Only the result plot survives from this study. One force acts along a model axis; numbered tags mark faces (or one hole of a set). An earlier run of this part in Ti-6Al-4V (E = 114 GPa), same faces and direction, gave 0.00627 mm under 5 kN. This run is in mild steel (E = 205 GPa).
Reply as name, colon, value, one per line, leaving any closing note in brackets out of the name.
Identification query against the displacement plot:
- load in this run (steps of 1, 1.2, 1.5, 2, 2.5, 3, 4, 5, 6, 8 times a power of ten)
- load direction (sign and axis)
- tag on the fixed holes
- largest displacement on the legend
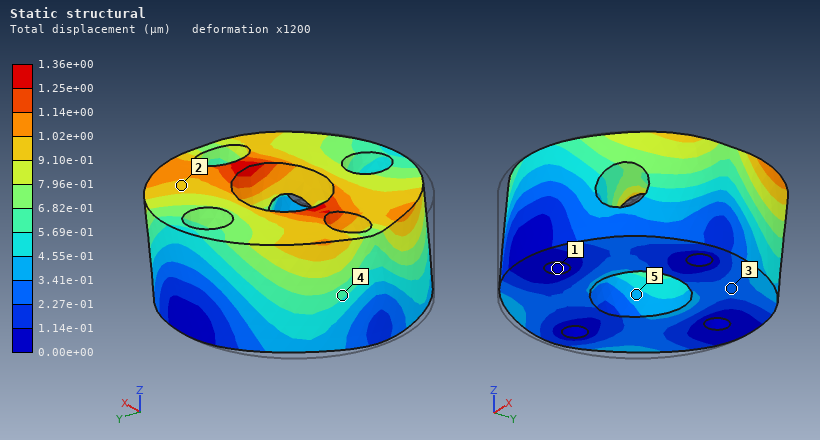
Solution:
load in this run: 2 kN
load direction: +X
tag on the fixed holes: 1
largest displacement on the legend: 1.36e+00 µm
